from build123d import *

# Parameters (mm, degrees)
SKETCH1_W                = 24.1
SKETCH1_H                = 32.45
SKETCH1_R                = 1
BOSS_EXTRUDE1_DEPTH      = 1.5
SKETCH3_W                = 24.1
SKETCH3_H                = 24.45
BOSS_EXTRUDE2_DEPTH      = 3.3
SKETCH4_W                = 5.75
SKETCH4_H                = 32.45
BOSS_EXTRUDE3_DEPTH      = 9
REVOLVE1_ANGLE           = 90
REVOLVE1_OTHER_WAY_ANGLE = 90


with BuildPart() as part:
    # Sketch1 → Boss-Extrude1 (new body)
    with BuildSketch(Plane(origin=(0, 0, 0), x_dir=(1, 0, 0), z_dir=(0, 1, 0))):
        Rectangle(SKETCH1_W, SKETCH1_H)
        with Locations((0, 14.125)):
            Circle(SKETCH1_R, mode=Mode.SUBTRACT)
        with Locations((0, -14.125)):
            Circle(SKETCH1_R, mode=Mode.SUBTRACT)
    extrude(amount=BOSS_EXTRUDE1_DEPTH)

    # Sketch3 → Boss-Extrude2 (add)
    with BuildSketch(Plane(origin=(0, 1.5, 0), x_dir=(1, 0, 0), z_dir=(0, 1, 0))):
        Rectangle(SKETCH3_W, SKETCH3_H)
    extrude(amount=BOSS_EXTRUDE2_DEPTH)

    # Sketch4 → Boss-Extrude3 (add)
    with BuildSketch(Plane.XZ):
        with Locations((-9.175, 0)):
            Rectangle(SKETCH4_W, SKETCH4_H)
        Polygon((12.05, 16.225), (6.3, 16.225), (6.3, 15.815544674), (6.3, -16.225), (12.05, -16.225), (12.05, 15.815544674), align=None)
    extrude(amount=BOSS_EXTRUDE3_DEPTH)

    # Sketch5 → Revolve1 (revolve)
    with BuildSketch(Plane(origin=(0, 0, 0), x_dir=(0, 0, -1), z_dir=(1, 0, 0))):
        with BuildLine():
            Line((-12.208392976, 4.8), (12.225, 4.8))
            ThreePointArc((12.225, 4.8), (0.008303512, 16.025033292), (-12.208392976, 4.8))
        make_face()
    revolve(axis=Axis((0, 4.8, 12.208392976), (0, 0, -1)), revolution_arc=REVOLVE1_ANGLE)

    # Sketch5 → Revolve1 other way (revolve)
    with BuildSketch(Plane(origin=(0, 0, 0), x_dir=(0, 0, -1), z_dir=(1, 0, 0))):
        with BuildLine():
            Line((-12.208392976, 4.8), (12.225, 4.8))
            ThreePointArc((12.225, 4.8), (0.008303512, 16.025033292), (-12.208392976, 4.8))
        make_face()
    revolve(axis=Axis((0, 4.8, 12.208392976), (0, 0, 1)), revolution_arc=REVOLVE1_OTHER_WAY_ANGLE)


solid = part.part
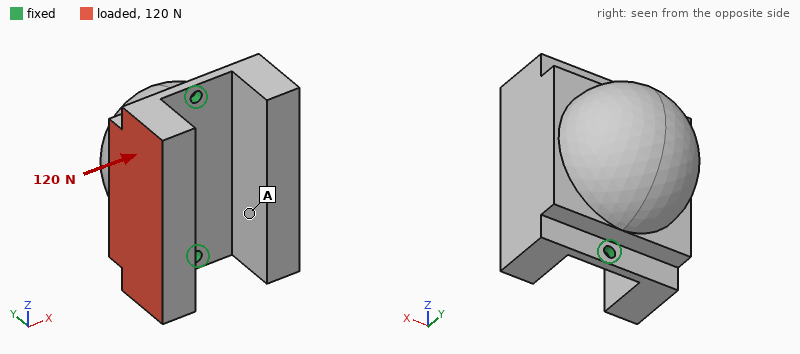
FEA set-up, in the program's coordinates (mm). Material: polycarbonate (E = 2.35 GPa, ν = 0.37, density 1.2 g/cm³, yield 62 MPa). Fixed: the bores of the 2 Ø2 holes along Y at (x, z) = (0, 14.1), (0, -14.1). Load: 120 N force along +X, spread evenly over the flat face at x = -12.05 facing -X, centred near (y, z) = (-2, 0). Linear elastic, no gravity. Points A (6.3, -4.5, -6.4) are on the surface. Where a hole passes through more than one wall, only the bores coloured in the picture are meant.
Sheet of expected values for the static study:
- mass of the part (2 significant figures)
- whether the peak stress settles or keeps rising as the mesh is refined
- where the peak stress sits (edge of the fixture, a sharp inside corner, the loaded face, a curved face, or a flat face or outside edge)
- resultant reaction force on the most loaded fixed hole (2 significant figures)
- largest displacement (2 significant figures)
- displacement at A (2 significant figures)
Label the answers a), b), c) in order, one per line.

a) 12 g
b) keeps rising
c) edge of the fixture
d) 61 N
e) 0.51 mm
f) 0.25 mm
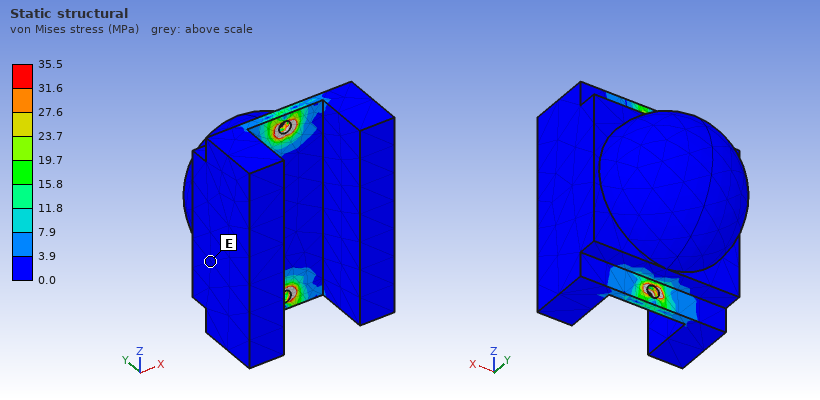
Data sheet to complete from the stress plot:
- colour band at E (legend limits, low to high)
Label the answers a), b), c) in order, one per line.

a) 0.0 to 3.9 MPa
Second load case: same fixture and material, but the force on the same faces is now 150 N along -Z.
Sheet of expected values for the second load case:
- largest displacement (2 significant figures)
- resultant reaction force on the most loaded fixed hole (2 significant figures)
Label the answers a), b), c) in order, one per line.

a) 82 µm
b) 100 N
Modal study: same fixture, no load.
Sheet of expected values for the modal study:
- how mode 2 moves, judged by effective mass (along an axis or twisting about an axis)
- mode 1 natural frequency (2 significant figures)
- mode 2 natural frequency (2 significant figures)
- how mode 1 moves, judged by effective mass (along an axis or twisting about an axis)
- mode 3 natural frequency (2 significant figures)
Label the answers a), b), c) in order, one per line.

a) along Y
b) 560 Hz
c) 2700 Hz
d) twisting about Z
e) 3300 Hz
